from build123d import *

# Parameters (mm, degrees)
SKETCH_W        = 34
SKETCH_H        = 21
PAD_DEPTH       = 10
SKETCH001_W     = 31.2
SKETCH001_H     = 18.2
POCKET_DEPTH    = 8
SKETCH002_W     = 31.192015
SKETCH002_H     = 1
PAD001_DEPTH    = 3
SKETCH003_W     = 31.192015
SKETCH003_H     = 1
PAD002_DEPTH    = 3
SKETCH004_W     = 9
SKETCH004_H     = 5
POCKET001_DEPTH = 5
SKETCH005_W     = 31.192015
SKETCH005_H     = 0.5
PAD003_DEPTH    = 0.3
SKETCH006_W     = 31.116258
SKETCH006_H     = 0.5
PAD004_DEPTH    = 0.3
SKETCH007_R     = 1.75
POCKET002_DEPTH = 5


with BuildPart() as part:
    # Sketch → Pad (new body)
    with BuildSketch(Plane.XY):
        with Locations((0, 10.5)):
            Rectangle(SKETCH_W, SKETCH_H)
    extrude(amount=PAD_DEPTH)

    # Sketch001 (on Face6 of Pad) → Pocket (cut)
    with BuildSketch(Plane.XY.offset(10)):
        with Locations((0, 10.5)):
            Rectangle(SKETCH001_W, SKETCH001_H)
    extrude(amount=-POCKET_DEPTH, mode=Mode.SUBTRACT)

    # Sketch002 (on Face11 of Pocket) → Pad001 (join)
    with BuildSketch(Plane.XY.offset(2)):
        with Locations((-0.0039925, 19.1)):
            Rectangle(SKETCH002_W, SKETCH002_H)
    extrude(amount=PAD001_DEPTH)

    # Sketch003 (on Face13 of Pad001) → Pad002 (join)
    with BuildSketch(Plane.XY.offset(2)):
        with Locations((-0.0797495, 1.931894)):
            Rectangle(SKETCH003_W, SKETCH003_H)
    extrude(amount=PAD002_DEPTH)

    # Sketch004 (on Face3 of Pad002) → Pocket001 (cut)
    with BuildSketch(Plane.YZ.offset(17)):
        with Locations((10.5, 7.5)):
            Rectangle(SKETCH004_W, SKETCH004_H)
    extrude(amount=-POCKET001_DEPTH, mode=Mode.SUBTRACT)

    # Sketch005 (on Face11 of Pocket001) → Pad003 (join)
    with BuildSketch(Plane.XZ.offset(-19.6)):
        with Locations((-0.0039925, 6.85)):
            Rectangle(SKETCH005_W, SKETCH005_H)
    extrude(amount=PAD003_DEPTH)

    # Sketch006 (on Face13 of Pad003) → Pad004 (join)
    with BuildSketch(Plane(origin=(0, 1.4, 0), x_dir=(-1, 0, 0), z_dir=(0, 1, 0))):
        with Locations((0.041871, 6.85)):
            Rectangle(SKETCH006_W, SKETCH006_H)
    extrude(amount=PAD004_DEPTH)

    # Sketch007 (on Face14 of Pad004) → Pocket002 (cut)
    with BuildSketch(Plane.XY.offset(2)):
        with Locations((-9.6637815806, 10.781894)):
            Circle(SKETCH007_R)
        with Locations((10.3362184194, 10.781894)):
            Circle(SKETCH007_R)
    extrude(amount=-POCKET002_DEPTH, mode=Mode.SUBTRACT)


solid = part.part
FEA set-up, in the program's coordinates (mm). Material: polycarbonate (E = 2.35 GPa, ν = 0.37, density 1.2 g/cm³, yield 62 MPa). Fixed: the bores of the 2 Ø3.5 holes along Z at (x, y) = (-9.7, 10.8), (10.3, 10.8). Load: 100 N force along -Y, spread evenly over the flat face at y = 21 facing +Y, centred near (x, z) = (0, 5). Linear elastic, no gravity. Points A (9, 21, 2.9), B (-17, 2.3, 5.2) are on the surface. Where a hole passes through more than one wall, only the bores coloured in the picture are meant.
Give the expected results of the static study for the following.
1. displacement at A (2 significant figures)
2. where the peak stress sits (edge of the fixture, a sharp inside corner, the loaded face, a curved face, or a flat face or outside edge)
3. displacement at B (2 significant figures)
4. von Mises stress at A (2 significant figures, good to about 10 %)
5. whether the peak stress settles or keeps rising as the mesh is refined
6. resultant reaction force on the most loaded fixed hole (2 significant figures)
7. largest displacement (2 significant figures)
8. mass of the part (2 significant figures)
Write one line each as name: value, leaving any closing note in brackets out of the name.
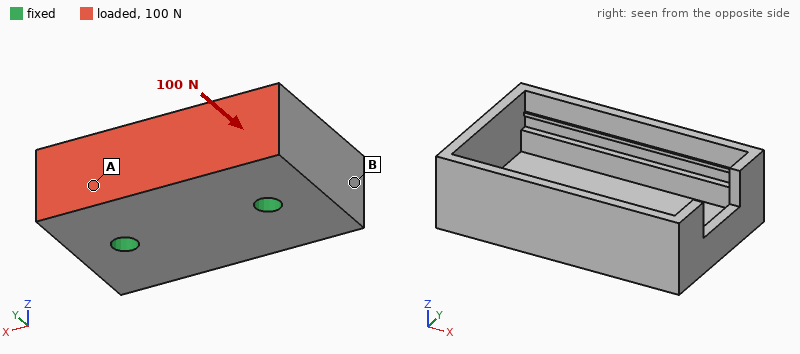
displacement at A: 0.20 mm
where the peak stress sits: edge of the fixture
displacement at B: 0.12 mm
von Mises stress at A: 6.1 MPa
whether the peak stress settles or keeps rising as the mesh is refined: keeps rising
resultant reaction force on the most loaded fixed hole: 53 N
largest displacement: 0.46 mm
mass of the part: 3.2 g
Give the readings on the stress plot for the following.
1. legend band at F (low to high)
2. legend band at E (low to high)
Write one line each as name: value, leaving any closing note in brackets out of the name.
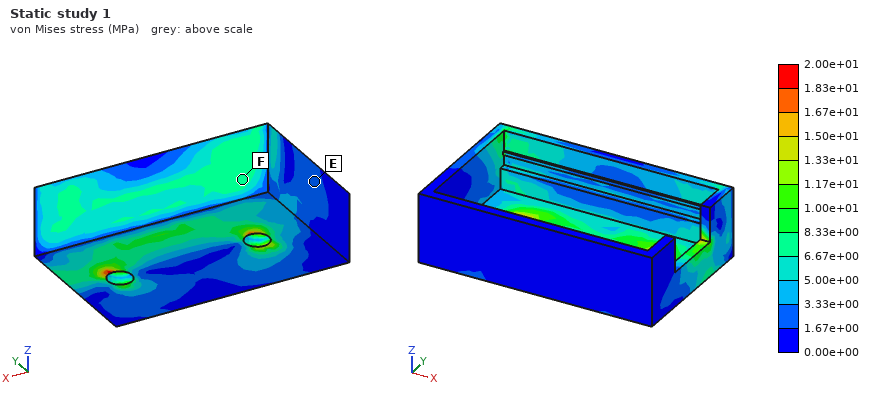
legend band at F: 6.67e+00 to 8.33e+00 MPa
legend band at E: 1.67e+00 to 3.33e+00 MPa
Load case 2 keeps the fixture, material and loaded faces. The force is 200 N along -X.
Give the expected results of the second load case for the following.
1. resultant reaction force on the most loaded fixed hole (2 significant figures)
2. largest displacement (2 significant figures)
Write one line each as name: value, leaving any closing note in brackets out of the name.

resultant reaction force on the most loaded fixed hole: 140 N
largest displacement: 0.33 mm
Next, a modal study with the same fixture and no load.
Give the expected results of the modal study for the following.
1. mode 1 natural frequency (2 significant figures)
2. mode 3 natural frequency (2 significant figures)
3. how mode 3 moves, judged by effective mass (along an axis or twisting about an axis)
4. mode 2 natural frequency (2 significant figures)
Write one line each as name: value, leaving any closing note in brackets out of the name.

mode 1 natural frequency: 2000 Hz
mode 3 natural frequency: 3200 Hz
how mode 3 moves, judged by effective mass: along Z
mode 2 natural frequency: 2500 Hz
